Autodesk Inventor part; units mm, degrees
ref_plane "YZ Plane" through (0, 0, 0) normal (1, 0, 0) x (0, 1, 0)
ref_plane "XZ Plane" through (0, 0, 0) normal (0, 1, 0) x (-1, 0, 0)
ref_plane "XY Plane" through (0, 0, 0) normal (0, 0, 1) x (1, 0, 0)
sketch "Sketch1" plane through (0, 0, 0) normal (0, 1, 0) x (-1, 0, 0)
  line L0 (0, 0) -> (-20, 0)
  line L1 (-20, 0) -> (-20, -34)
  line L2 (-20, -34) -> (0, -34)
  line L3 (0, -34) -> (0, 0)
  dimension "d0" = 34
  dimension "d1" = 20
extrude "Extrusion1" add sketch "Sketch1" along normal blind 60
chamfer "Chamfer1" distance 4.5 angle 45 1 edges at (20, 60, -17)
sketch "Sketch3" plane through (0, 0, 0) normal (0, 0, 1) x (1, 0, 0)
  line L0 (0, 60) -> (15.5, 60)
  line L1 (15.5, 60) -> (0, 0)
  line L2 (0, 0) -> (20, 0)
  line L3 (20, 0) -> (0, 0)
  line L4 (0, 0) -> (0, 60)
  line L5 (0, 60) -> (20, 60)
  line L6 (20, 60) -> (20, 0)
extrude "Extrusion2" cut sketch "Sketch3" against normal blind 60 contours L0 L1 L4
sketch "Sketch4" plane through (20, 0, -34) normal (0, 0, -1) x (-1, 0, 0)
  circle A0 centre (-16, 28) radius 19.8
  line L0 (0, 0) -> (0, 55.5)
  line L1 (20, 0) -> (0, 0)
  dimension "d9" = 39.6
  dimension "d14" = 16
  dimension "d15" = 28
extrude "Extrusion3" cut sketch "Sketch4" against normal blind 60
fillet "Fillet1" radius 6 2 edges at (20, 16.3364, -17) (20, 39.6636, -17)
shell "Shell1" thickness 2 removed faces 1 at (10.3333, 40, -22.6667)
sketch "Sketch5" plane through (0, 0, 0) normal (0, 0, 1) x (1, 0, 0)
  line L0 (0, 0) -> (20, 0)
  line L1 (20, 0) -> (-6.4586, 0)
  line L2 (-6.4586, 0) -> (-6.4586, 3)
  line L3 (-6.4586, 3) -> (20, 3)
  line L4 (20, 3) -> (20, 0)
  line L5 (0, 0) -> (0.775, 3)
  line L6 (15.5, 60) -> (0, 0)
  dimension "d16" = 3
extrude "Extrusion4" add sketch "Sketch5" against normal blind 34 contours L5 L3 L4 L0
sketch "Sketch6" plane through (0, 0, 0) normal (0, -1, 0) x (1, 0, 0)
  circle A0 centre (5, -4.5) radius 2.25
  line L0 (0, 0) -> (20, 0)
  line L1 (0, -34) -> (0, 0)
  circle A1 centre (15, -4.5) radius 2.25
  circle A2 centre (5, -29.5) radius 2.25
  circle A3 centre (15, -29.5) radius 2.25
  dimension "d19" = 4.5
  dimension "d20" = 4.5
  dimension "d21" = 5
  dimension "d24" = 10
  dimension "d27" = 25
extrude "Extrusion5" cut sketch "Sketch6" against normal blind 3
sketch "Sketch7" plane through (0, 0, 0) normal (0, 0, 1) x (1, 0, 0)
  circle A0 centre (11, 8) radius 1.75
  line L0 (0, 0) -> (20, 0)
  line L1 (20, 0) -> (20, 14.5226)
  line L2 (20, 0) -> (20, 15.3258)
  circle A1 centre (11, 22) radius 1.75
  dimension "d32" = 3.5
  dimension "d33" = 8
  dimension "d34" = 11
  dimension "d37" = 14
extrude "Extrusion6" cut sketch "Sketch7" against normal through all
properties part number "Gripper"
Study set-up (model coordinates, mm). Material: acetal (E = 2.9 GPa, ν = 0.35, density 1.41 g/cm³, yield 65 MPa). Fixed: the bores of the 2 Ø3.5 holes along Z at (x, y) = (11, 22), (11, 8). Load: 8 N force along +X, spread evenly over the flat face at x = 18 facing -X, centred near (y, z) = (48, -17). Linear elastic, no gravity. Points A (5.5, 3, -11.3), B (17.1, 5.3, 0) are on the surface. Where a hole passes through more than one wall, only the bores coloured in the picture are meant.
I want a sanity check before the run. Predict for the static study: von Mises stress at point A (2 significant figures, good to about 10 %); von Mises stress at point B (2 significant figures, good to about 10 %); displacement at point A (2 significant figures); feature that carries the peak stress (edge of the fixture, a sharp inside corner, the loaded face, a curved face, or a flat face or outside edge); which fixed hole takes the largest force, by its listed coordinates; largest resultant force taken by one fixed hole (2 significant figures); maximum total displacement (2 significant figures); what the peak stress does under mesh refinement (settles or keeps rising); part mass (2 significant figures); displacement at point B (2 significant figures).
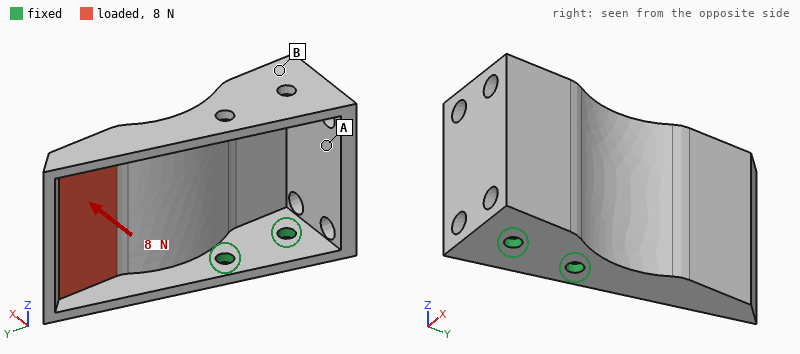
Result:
1.7 MPa
0.80 MPa
0.16 mm
edge of the fixture
(11, 22)
17 N
0.83 mm
keeps rising
11 g
0.19 mm
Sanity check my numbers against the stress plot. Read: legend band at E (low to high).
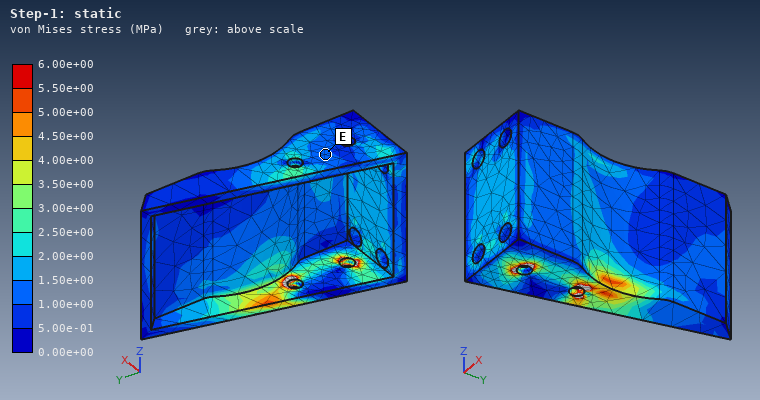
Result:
1.00e+00 to 1.50e+00 MPa
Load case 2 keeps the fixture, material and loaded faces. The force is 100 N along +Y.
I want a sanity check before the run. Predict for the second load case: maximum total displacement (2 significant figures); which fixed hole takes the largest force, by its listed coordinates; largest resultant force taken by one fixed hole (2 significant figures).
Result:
0.80 mm
(11, 22)
110 N
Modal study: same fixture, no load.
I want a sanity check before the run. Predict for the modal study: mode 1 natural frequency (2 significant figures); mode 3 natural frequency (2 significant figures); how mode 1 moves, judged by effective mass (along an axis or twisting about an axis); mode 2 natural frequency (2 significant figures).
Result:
280 Hz
830 Hz
along X
510 Hz
